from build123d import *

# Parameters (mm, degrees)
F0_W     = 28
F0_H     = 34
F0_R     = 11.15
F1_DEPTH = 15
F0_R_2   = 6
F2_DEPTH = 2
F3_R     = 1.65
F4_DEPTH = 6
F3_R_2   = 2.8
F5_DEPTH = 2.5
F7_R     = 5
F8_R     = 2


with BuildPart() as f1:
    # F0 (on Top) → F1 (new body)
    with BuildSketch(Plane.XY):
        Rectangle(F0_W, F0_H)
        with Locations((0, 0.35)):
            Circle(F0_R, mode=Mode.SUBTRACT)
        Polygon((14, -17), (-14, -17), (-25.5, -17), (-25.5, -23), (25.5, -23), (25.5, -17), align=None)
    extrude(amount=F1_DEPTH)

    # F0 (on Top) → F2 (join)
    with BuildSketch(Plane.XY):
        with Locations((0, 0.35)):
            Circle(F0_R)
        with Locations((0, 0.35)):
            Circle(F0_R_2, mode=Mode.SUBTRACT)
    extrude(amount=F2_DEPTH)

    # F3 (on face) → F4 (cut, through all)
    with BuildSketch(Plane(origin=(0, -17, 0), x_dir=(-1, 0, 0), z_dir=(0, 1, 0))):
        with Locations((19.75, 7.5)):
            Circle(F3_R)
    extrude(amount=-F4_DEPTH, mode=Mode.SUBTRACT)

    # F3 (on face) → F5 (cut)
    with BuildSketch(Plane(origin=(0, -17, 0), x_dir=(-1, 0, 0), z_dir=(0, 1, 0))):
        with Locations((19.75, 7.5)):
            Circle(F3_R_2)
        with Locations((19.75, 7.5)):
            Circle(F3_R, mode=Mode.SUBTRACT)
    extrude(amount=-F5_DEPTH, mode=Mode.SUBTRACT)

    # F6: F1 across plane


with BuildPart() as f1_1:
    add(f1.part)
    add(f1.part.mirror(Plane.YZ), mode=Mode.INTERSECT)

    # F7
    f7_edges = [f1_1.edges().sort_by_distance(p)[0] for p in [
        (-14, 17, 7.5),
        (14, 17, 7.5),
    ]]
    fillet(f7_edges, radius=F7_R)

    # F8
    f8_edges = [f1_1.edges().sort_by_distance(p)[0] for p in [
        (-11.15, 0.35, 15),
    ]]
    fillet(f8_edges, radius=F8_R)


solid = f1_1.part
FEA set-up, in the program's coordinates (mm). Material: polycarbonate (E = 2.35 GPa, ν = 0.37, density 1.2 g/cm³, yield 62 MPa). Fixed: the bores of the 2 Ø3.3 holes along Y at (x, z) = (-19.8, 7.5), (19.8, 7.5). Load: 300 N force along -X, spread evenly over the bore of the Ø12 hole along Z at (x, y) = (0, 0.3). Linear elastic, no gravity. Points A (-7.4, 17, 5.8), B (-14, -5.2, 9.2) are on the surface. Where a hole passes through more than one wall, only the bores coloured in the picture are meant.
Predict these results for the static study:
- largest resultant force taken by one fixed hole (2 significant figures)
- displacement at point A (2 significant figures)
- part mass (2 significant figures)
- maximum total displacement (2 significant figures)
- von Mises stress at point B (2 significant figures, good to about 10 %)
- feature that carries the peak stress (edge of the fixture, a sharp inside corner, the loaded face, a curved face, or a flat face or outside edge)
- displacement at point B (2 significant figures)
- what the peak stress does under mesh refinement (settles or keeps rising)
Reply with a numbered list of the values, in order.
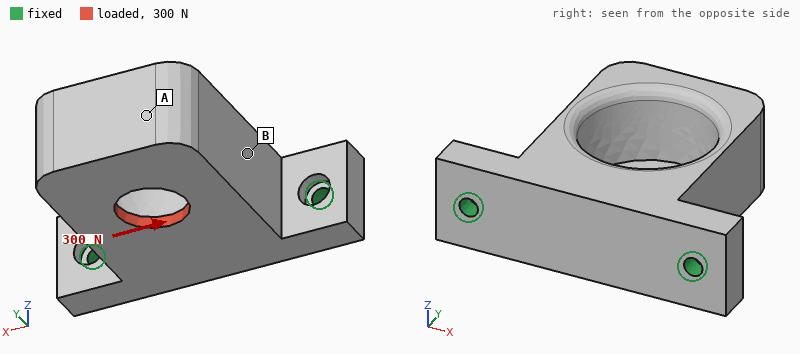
1. 240 N
2. 0.24 mm
3. 16 g
4. 0.26 mm
5. 4.8 MPa
6. edge of the fixture
7. 0.093 mm
8. keeps rising
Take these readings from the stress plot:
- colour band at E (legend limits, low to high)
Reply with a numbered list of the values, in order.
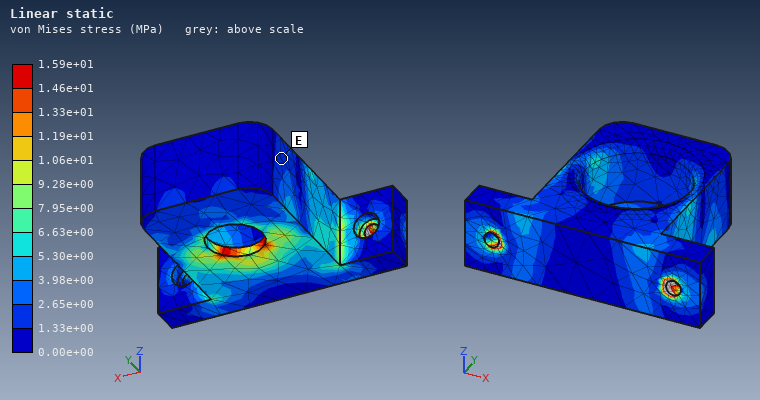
1. 1.33e+00 to 2.65e+00 MPa
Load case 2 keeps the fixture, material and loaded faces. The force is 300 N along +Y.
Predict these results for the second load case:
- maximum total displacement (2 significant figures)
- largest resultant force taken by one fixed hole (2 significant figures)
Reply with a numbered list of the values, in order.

1. 0.77 mm
2. 180 N
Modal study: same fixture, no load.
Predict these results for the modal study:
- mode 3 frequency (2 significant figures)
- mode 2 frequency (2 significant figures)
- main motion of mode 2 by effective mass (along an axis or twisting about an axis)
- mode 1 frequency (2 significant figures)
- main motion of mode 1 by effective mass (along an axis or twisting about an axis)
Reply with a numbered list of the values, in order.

1. 3200 Hz
2. 1800 Hz
3. along X
4. 640 Hz
5. along Z
